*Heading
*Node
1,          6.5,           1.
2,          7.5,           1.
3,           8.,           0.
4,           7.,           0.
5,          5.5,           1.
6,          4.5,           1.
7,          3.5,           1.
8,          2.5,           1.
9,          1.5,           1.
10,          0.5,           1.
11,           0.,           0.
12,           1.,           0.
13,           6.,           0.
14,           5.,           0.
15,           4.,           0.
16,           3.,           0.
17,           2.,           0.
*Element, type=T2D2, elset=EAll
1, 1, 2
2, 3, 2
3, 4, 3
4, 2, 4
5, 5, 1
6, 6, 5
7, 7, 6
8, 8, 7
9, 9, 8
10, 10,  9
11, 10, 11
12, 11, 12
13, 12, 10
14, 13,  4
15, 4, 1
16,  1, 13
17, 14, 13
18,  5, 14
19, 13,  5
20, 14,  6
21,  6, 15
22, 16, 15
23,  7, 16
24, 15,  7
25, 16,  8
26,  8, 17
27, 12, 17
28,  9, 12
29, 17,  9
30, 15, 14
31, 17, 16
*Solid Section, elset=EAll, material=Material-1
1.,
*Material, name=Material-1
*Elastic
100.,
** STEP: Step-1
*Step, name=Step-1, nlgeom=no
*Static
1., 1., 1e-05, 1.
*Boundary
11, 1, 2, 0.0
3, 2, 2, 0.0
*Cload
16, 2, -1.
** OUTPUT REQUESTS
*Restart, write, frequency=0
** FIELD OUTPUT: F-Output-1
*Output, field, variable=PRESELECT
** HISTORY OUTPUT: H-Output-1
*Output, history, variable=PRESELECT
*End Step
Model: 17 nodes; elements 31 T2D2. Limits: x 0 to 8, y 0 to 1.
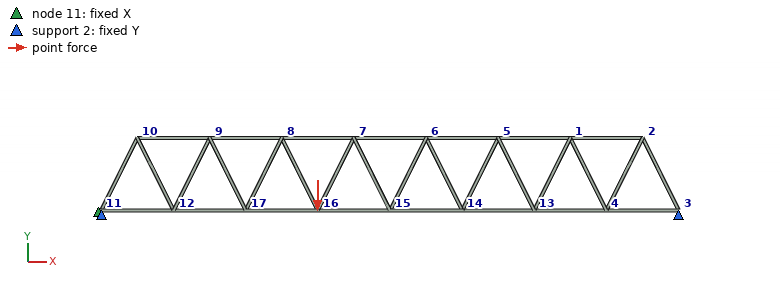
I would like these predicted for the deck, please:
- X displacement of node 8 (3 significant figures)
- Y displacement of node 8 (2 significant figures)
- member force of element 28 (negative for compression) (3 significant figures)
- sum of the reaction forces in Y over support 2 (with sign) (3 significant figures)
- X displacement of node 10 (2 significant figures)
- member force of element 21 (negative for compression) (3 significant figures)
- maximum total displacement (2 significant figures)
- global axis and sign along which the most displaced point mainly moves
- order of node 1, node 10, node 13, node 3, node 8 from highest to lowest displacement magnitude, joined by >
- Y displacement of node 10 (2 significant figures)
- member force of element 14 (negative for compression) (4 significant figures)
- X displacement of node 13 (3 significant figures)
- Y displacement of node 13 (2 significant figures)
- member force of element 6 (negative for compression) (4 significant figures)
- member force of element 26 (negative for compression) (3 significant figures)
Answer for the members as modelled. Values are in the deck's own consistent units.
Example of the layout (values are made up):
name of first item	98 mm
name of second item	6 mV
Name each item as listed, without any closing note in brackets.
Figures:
X displacement of node 8	0.0625
Y displacement of node 8	-0.22
member force of element 28 (negative for compression)	-0.699
sum of the reaction forces in Y over support 2 (with sign)	1.00
X displacement of node 10	0.081
member force of element 21 (negative for compression)	0.419
maximum total displacement	0.25
global axis and sign along which the most displaced point mainly moves	-Y
order of node 1, node 10, node 13, node 3, node 8 from highest to lowest displacement magnitude, joined by >	node 8 > node 13 > node 1 > node 10 > node 3
Y displacement of node 10	-0.049
member force of element 14 (negative for compression)	0.5625
X displacement of node 13	0.0675
Y displacement of node 13	-0.15
member force of element 6 (negative for compression)	-1.125
member force of element 26 (negative for compression)	-0.699
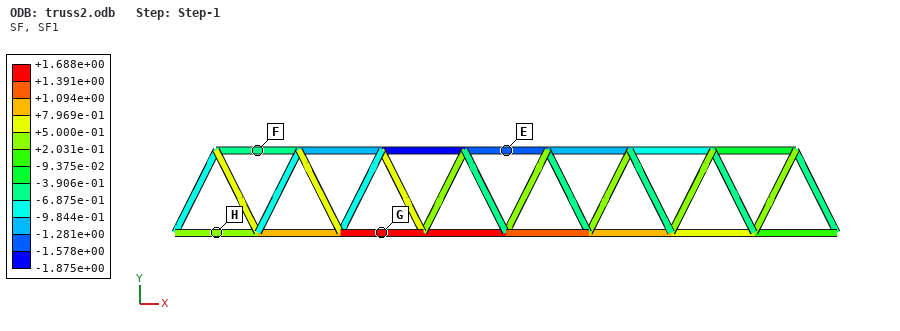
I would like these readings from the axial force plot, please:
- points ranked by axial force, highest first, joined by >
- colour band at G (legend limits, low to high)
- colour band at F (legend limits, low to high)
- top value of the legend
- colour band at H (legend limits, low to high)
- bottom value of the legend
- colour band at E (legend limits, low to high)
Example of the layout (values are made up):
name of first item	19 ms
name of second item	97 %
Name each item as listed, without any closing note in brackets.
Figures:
points ranked by axial force, highest first, joined by >	G > H > F > E
colour band at G	+1.391e+00 to +1.688e+00
colour band at F	-6.875e-01 to -3.906e-01
top value of the legend	+1.688e+00
colour band at H	+2.031e-01 to +5.000e-01
bottom value of the legend	-1.875e+00
colour band at E	-1.578e+00 to -1.281e+00
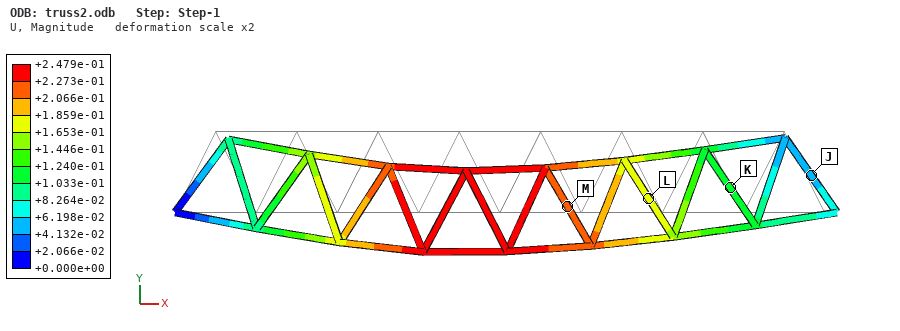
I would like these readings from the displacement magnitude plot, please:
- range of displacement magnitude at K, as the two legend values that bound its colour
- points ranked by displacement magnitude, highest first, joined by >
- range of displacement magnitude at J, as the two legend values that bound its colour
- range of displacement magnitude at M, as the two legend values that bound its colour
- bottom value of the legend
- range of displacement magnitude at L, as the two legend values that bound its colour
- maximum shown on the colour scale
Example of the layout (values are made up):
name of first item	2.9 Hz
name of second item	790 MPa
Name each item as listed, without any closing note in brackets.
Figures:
range of displacement magnitude at K, as the two legend values that bound its colour	+1.033e-01 to +1.240e-01
points ranked by displacement magnitude, highest first, joined by >	M > L > K > J
range of displacement magnitude at J, as the two legend values that bound its colour	+4.132e-02 to +6.198e-02
range of displacement magnitude at M, as the two legend values that bound its colour	+2.066e-01 to +2.273e-01
bottom value of the legend	+0.000e+00
range of displacement magnitude at L, as the two legend values that bound its colour	+1.653e-01 to +1.859e-01
maximum shown on the colour scale	+2.479e-01
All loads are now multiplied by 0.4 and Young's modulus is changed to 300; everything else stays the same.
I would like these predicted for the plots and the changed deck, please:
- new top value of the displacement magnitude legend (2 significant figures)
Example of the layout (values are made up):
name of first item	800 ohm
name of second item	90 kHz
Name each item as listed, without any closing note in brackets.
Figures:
new top value of the displacement magnitude legend	0.033
